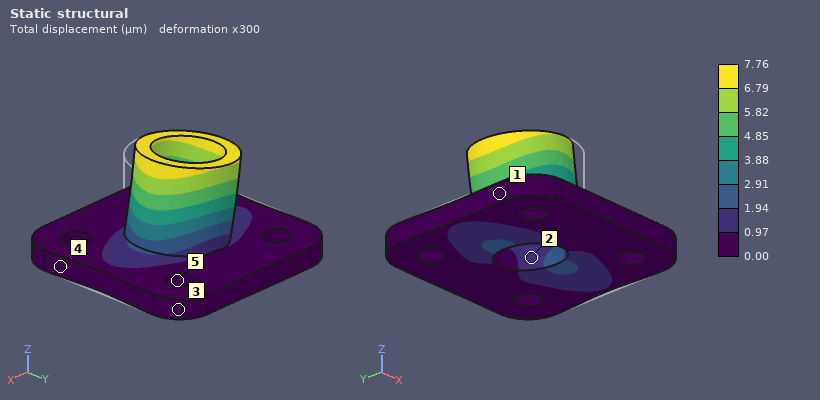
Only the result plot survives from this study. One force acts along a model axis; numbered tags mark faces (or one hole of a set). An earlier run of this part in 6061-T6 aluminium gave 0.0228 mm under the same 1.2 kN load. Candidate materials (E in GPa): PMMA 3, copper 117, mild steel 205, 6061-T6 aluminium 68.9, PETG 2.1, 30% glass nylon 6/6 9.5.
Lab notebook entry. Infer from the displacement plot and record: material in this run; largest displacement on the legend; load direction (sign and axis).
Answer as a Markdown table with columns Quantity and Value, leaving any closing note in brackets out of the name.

| Quantity | Value |
|---|---|
| material in this run | mild steel |
| largest displacement on the legend | 7.76 µm |
| load direction | -X |
